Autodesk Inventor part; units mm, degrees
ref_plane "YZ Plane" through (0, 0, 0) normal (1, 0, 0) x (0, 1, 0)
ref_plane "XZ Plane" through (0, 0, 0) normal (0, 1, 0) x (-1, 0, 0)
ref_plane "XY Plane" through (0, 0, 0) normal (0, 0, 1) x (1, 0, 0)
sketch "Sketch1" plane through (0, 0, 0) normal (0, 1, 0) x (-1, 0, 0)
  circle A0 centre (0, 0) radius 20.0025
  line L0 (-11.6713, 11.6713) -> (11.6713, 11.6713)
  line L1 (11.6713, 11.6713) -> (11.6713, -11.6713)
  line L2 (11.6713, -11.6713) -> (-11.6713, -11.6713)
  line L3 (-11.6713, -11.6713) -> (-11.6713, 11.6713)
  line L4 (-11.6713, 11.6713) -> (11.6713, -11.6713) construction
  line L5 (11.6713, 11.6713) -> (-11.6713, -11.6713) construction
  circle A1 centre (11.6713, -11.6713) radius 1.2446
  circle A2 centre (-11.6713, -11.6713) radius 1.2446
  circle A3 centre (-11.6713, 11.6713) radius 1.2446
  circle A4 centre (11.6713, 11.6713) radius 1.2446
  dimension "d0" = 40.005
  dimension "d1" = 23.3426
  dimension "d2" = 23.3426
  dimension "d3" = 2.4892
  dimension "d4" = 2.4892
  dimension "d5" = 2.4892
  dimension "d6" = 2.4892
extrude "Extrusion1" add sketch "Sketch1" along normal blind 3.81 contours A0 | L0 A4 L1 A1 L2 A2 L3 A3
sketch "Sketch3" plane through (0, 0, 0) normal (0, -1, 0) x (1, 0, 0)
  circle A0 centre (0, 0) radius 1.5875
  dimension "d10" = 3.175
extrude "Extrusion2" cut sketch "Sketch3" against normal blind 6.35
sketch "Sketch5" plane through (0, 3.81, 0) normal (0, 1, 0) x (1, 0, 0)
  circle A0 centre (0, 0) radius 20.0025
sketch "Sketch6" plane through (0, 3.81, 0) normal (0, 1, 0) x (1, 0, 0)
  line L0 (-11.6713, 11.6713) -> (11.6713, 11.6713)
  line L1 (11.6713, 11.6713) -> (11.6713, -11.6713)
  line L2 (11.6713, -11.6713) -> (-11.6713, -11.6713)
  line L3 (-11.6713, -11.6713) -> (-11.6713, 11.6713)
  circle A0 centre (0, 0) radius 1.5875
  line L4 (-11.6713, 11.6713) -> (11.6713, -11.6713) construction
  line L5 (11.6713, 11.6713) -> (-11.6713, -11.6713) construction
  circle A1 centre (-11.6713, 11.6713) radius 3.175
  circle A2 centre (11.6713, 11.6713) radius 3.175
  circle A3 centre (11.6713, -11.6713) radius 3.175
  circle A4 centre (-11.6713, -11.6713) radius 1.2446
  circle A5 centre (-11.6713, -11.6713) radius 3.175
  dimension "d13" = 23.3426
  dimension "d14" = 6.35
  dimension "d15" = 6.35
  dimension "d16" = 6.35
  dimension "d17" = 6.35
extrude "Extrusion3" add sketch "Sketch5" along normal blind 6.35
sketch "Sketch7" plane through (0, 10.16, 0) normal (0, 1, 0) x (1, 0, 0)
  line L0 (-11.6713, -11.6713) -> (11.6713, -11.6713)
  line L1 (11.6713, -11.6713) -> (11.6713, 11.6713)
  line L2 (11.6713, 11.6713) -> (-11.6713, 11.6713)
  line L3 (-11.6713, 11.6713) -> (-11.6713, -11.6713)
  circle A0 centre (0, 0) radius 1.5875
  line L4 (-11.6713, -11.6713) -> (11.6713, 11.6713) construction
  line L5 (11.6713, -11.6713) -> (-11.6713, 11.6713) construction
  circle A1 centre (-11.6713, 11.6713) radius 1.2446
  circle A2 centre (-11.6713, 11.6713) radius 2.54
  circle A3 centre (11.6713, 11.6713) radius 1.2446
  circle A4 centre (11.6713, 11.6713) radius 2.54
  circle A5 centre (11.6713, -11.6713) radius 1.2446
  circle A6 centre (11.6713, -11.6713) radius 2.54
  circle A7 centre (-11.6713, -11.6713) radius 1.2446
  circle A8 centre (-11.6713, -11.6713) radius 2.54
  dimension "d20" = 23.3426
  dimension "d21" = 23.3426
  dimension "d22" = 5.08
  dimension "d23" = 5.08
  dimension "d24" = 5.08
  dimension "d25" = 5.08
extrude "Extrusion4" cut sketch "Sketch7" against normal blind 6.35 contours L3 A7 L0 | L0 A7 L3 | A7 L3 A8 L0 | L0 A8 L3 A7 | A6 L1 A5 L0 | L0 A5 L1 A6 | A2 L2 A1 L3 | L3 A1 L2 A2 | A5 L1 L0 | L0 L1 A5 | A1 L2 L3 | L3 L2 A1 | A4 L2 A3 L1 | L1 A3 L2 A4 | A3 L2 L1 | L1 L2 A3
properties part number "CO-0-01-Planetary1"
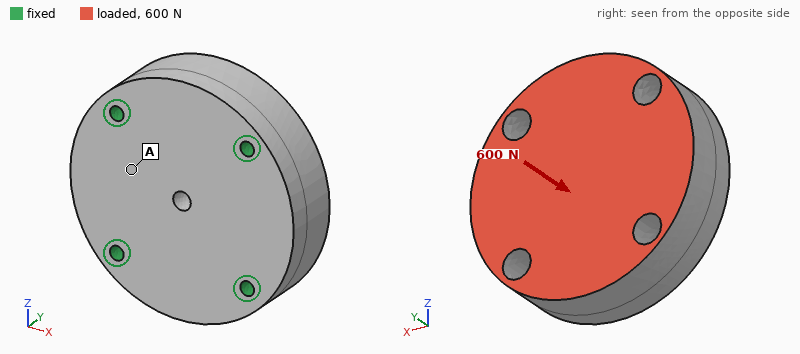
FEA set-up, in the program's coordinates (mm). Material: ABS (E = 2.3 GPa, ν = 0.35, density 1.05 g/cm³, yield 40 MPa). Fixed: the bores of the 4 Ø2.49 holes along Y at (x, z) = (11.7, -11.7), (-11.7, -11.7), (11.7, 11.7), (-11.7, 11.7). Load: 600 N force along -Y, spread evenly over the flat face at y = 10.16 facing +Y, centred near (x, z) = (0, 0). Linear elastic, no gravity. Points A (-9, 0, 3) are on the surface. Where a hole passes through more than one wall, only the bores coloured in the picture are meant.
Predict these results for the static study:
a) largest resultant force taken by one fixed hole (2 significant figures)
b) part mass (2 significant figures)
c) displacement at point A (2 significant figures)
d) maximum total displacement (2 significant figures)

160 N
13 g
19 µm
23 µm
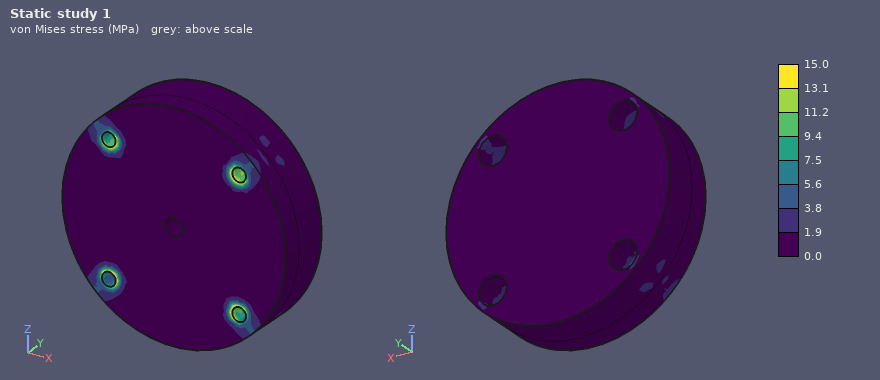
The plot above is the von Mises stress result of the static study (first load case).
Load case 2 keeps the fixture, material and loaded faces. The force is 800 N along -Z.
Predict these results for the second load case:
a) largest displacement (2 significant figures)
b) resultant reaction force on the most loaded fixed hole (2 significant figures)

55 µm
240 N
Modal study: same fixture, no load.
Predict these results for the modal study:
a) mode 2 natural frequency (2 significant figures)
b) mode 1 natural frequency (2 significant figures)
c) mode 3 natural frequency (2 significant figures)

8400 Hz
8100 Hz
8400 Hz
